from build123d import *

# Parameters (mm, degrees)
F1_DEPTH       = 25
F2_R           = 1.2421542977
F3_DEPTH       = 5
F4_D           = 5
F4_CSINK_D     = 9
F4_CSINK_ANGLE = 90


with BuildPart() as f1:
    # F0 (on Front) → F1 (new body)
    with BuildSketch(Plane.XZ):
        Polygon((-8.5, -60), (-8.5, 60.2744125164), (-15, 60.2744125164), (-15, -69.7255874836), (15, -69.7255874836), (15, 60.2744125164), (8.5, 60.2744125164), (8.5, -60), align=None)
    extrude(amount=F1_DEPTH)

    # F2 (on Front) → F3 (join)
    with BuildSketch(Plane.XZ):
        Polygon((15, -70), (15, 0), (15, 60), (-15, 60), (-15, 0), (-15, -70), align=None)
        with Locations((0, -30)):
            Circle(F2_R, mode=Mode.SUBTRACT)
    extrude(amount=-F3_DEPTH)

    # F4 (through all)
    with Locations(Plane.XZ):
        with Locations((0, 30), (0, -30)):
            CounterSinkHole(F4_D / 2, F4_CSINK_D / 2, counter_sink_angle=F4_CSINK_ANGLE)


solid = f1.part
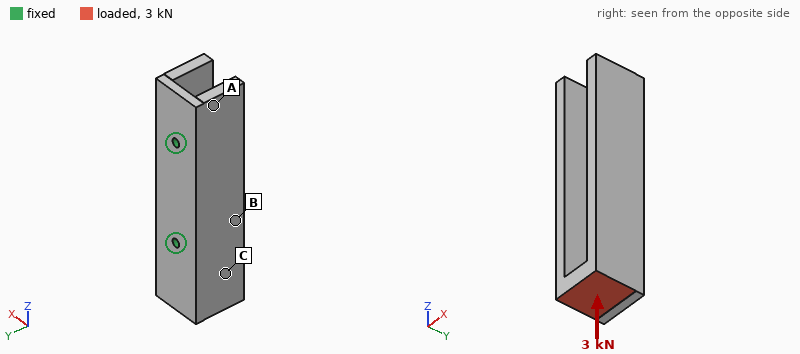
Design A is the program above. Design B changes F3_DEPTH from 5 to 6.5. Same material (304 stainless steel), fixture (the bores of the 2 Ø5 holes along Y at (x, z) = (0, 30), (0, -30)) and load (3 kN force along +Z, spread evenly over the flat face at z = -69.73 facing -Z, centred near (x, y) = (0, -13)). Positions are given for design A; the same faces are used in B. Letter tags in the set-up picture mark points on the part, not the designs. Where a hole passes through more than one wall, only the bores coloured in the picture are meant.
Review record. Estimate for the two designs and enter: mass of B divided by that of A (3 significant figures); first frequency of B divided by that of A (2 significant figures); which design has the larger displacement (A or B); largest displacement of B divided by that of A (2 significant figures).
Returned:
1.09
1.3
A
0.83
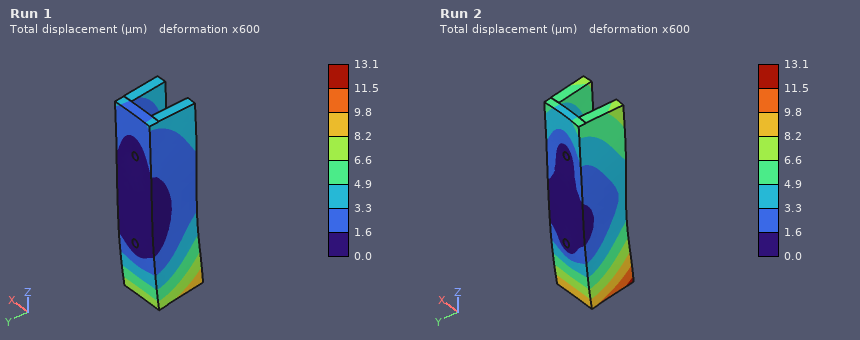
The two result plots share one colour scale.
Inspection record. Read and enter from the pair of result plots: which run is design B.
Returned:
Run 1
